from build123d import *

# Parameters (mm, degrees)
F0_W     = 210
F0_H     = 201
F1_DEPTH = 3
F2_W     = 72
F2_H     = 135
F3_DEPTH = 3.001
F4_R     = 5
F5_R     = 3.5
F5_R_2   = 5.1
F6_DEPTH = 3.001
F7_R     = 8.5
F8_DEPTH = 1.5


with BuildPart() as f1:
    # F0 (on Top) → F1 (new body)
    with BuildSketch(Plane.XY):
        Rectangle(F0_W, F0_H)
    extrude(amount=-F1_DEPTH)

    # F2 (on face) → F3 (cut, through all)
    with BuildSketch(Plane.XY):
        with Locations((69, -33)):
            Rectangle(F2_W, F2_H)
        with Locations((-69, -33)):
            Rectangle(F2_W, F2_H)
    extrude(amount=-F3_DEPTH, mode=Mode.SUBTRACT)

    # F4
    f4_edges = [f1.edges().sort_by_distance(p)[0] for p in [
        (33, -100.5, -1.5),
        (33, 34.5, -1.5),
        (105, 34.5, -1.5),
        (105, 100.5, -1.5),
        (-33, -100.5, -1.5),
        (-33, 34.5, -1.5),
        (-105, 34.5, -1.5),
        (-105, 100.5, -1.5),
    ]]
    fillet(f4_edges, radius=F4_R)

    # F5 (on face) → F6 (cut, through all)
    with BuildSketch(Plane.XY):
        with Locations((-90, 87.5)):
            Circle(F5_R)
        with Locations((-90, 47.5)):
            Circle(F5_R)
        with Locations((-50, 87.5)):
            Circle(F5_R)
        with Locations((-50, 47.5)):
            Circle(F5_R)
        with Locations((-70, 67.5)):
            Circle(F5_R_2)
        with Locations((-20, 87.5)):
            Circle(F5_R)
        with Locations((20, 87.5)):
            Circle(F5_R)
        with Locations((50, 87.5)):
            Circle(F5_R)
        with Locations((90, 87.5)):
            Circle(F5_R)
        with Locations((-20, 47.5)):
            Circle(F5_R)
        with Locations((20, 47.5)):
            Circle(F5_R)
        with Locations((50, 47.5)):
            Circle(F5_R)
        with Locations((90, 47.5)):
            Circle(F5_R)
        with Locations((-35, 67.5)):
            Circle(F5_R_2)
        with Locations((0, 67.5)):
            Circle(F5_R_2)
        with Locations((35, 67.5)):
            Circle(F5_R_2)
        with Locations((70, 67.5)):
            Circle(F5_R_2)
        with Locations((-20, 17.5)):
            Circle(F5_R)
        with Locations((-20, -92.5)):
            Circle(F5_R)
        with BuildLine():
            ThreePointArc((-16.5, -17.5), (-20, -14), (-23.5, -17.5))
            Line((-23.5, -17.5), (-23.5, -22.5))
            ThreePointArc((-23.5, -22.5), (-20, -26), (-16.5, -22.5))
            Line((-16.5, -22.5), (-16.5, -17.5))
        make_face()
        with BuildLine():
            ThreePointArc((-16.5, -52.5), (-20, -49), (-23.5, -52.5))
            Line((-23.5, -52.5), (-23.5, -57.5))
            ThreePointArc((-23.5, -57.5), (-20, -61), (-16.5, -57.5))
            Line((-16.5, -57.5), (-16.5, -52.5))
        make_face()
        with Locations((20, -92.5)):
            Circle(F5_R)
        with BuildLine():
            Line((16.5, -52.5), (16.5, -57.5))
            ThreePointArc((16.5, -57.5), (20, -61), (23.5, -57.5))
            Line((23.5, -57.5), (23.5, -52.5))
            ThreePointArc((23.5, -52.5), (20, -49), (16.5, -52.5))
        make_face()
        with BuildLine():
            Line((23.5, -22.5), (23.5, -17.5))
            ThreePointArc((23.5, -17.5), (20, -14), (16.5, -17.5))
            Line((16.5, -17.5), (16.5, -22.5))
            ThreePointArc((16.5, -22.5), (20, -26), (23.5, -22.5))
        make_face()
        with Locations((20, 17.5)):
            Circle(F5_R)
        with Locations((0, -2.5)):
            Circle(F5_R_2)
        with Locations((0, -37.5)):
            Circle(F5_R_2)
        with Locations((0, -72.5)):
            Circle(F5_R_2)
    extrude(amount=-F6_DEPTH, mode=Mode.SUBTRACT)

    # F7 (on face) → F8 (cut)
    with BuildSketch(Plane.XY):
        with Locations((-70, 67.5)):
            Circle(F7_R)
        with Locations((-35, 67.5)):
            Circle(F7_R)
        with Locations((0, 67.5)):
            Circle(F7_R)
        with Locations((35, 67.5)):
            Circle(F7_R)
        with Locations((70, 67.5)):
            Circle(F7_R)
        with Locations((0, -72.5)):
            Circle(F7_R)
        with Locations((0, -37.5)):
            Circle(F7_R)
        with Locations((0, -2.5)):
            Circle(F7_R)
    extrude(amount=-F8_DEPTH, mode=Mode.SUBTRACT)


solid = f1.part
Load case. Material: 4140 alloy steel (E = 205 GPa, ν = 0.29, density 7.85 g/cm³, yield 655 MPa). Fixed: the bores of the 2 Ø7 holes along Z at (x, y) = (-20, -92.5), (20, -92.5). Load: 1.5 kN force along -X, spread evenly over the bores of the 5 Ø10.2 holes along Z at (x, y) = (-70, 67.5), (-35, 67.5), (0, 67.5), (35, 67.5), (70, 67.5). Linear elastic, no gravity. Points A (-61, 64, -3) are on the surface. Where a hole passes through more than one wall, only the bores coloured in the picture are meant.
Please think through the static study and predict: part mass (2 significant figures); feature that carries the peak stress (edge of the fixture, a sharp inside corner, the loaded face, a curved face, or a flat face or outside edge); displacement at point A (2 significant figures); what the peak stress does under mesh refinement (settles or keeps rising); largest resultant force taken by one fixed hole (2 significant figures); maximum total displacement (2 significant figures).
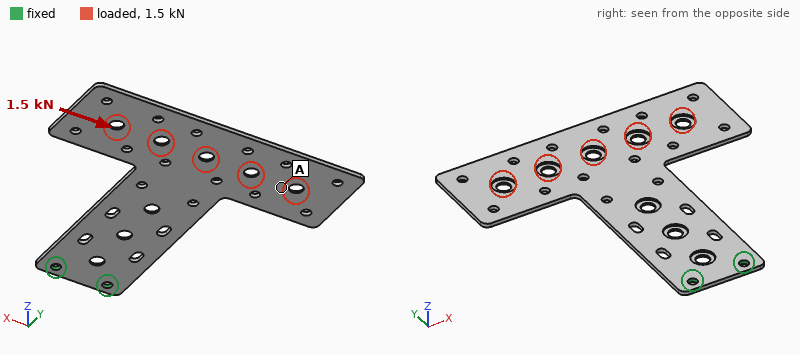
490 g
edge of the fixture
0.29 mm
keeps rising
5.4 kN
0.47 mm
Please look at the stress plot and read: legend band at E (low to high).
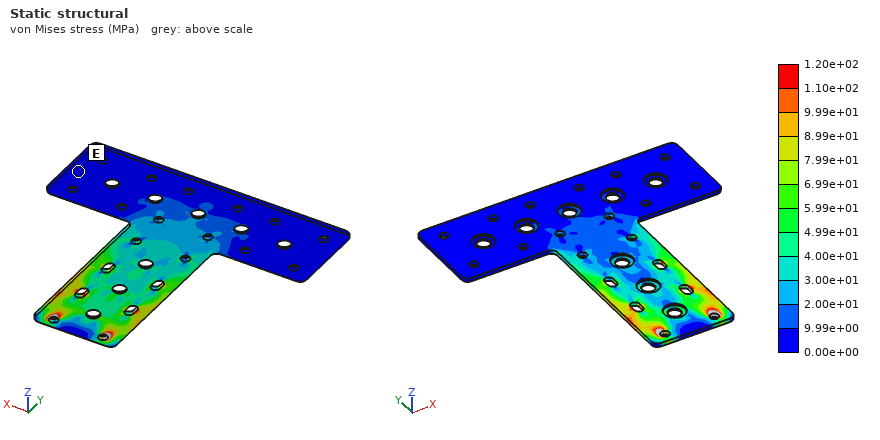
0.00e+00 to 9.99e+00 MPa
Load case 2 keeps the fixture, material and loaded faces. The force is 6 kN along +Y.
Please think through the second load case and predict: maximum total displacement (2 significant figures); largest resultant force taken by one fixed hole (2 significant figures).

2.9 mm
3.0 kN
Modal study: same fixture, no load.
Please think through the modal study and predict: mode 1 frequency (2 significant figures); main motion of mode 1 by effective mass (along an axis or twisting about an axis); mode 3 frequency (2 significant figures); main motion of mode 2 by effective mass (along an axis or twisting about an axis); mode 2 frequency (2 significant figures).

38 Hz
along Z
330 Hz
twisting about Y
82 Hz
